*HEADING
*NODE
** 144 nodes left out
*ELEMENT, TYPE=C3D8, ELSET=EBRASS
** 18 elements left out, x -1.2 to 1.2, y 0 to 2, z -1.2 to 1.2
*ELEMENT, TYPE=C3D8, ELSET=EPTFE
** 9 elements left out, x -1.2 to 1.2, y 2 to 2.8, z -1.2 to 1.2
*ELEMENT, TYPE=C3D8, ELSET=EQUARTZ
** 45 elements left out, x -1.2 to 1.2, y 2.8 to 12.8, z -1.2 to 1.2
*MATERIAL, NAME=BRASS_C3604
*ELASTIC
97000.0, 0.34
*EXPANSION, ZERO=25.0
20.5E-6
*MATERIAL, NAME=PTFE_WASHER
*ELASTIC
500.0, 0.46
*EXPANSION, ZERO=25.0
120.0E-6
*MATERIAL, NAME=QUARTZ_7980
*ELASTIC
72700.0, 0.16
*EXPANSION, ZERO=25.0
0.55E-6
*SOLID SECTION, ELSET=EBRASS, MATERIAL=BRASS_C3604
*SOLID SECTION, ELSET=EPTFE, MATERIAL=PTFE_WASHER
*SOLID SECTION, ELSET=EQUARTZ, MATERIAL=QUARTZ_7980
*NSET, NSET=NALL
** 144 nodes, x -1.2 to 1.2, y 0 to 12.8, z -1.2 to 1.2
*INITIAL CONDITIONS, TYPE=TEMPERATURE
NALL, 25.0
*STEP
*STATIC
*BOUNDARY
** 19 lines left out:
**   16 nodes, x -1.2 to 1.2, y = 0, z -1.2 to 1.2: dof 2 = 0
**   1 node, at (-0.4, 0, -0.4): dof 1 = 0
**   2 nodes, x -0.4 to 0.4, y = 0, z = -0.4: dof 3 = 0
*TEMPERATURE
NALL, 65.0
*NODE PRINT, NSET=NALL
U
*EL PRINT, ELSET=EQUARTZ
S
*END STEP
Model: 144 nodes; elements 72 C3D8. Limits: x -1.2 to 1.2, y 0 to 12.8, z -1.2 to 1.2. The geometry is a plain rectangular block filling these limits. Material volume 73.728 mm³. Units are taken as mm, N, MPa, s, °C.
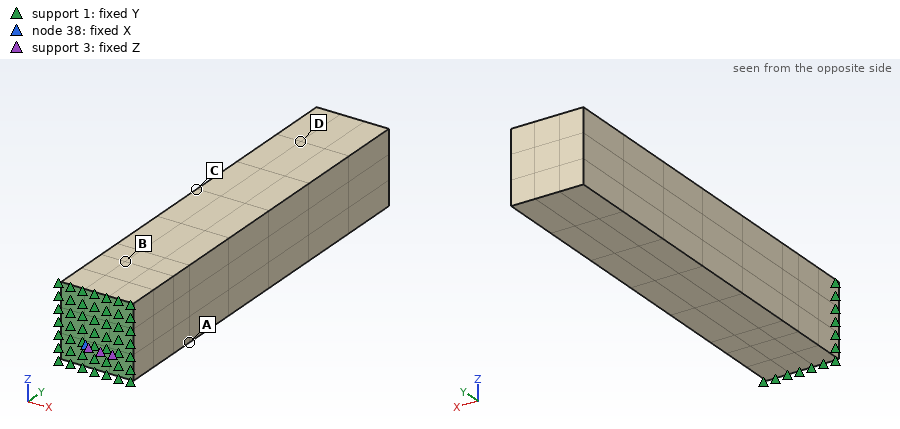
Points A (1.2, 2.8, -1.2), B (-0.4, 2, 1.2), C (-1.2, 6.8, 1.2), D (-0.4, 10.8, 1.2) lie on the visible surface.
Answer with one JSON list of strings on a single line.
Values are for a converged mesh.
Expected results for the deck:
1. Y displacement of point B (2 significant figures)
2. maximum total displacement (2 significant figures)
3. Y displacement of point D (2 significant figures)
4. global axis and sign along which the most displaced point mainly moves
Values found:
["0.0016 mm", "0.0093 mm", "0.0092 mm", "+Y"]
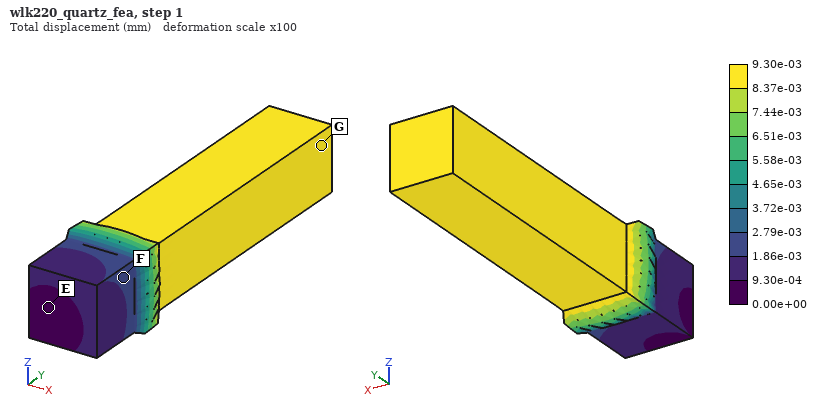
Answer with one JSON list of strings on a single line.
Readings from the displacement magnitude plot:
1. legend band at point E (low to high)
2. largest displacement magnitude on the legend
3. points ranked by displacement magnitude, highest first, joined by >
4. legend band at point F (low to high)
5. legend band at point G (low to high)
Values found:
["0.00e+00 to 9.30e-04 mm", "9.30e-03 mm", "G > F > E", "1.86e-03 to 2.79e-03 mm", "8.37e-03 to 9.30e-03 mm"]
